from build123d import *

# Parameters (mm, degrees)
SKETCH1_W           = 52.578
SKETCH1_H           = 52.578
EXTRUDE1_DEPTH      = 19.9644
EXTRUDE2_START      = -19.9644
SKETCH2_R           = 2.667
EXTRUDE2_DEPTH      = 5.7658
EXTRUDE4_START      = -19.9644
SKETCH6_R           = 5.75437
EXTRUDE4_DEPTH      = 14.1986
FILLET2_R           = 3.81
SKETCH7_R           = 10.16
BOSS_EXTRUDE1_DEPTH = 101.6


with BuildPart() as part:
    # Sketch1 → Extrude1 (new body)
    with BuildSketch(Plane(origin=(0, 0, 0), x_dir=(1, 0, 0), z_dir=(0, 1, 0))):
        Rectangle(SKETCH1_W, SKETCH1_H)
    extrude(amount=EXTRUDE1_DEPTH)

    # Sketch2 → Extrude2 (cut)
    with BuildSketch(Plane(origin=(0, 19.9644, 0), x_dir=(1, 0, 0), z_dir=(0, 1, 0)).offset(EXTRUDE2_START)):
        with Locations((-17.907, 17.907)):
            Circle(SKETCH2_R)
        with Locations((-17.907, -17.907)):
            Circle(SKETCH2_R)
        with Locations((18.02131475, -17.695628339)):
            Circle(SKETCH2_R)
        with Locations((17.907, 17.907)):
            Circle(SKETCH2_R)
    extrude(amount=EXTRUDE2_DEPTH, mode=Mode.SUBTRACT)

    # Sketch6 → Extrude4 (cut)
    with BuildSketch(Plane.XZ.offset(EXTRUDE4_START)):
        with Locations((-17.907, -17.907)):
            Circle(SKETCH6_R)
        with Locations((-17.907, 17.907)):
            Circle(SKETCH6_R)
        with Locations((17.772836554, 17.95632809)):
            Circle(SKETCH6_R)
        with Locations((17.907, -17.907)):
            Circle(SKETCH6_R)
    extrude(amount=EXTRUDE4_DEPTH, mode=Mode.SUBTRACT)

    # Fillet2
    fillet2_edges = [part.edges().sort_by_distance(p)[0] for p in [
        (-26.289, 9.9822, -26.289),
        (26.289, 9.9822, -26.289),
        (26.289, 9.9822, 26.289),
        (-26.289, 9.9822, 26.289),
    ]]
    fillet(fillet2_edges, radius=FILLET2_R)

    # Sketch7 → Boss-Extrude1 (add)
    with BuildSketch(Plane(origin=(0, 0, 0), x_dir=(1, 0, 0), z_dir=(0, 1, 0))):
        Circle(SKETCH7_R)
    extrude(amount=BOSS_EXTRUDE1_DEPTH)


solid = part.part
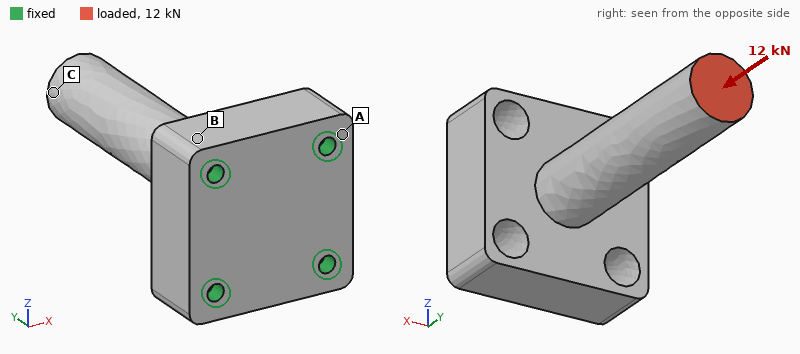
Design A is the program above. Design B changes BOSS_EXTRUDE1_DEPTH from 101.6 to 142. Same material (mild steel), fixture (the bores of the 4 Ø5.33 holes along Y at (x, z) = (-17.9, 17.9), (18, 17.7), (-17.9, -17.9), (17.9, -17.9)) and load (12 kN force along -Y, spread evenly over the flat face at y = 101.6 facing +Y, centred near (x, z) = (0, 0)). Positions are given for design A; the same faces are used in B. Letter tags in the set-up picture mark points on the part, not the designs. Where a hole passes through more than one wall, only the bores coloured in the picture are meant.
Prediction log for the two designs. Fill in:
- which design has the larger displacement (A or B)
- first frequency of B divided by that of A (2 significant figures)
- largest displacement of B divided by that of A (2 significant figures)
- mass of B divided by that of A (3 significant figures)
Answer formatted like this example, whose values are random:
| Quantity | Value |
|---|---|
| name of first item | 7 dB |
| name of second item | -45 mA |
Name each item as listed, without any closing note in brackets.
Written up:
| Quantity | Value |
|---|---|
| which design has the larger displacement | B |
| first frequency of B divided by that of A | 0.48 |
| largest displacement of B divided by that of A | 1.4 |
| mass of B divided by that of A | 1.17 |
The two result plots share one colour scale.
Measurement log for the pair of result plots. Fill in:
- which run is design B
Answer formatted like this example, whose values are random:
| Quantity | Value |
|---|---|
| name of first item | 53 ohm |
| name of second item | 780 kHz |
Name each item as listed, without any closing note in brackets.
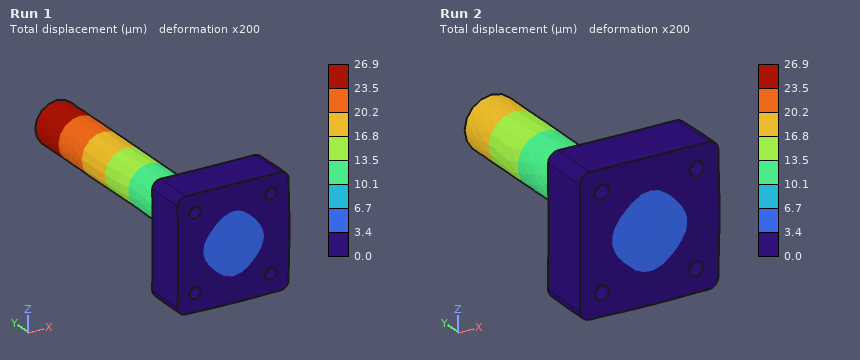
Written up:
| Quantity | Value |
|---|---|
| which run is design B | Run 1 |
